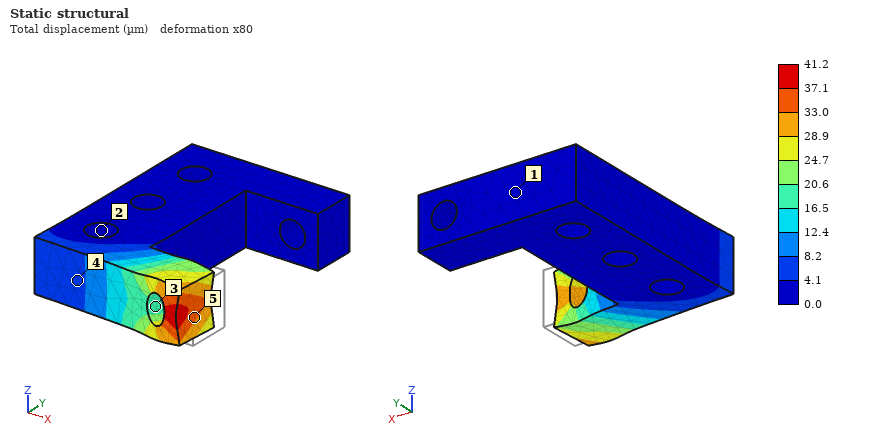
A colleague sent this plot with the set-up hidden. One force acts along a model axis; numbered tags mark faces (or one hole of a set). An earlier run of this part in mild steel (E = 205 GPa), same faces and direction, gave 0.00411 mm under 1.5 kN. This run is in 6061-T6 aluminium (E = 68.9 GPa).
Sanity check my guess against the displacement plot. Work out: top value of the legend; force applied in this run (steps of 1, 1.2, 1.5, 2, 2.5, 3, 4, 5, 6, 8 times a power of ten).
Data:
41.2 µm
5 kN
